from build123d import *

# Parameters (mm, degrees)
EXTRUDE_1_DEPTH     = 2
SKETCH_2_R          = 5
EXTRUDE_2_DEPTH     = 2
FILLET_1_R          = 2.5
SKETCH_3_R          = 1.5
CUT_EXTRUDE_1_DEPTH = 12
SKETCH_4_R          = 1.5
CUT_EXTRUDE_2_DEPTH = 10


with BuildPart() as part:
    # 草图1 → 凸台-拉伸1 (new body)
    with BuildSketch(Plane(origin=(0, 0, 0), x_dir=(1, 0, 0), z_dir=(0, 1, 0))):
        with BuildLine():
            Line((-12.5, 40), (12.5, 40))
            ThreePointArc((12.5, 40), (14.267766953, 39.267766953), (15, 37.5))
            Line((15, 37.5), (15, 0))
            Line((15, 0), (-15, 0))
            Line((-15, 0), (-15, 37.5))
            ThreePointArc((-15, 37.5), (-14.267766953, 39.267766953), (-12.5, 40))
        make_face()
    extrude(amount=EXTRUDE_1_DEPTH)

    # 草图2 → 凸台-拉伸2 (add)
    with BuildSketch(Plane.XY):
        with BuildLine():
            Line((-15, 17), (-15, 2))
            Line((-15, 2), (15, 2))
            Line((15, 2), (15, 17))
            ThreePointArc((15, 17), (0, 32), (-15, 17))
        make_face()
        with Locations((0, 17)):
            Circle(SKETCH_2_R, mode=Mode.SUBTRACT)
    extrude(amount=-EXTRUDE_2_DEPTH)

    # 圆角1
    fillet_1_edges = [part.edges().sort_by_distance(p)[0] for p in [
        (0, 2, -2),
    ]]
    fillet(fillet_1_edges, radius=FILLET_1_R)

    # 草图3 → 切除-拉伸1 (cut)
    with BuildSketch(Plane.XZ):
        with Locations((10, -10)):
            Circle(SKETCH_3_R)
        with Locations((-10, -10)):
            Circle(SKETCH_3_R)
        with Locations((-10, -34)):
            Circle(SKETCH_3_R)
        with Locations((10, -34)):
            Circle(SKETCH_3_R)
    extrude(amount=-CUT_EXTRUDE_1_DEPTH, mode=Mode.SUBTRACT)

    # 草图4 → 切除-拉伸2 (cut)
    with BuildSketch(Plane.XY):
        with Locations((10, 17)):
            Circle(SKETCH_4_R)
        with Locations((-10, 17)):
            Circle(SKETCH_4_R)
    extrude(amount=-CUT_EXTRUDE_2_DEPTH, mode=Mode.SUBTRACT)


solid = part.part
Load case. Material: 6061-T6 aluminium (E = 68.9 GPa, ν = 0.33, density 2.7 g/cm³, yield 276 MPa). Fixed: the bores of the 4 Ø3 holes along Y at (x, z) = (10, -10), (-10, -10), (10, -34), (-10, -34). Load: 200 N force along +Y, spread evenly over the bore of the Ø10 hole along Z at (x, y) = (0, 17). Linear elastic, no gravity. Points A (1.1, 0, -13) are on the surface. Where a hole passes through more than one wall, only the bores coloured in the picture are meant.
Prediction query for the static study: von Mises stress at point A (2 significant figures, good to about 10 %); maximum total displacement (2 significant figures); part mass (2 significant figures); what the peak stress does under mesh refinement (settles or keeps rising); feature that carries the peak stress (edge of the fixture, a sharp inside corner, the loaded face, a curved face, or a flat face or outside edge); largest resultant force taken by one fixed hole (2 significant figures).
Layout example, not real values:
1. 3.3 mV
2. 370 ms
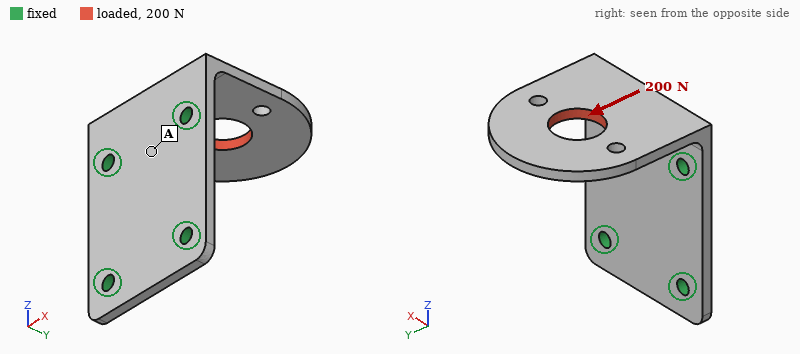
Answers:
1. 15 MPa
2. 0.17 mm
3. 10 g
4. keeps rising
5. edge of the fixture
6. 100 N
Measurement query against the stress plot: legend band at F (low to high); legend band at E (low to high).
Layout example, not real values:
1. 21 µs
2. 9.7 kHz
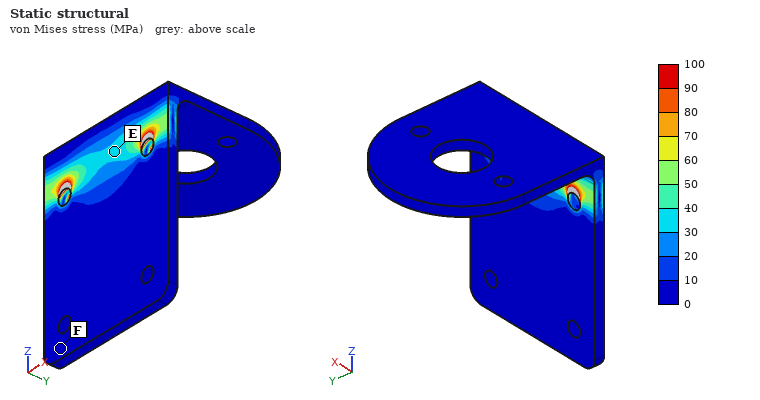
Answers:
1. 0 to 10 MPa
2. 30 to 40 MPa
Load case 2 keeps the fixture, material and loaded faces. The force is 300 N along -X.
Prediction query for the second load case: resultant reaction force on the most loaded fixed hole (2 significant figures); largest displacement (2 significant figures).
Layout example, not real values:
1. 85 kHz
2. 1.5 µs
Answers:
1. 290 N
2. 0.12 mm
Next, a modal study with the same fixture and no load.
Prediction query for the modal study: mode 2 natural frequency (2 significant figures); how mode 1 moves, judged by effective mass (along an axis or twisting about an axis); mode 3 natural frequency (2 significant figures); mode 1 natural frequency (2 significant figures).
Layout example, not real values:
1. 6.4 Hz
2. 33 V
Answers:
1. 4100 Hz
2. along Z
3. 6100 Hz
4. 1600 Hz
